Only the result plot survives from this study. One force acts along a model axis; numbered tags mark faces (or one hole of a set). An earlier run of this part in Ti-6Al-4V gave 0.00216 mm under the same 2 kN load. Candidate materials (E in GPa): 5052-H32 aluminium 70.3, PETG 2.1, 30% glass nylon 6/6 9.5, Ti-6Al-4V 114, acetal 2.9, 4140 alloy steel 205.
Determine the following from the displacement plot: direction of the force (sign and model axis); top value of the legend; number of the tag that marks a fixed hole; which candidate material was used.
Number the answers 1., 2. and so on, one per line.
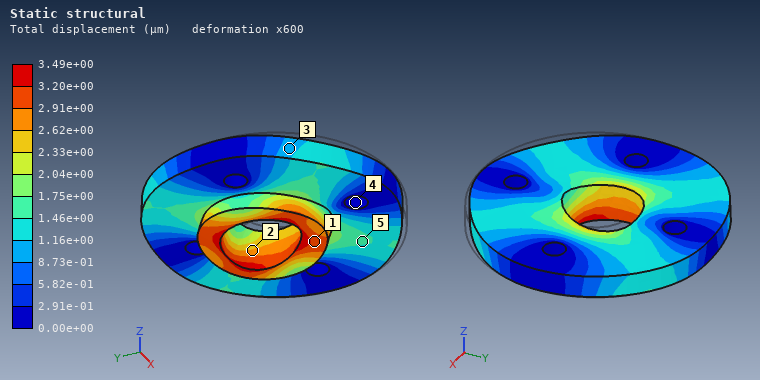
1. +Y
2. 3.49e+00 µm
3. 4
4. 5052-H32 aluminium
